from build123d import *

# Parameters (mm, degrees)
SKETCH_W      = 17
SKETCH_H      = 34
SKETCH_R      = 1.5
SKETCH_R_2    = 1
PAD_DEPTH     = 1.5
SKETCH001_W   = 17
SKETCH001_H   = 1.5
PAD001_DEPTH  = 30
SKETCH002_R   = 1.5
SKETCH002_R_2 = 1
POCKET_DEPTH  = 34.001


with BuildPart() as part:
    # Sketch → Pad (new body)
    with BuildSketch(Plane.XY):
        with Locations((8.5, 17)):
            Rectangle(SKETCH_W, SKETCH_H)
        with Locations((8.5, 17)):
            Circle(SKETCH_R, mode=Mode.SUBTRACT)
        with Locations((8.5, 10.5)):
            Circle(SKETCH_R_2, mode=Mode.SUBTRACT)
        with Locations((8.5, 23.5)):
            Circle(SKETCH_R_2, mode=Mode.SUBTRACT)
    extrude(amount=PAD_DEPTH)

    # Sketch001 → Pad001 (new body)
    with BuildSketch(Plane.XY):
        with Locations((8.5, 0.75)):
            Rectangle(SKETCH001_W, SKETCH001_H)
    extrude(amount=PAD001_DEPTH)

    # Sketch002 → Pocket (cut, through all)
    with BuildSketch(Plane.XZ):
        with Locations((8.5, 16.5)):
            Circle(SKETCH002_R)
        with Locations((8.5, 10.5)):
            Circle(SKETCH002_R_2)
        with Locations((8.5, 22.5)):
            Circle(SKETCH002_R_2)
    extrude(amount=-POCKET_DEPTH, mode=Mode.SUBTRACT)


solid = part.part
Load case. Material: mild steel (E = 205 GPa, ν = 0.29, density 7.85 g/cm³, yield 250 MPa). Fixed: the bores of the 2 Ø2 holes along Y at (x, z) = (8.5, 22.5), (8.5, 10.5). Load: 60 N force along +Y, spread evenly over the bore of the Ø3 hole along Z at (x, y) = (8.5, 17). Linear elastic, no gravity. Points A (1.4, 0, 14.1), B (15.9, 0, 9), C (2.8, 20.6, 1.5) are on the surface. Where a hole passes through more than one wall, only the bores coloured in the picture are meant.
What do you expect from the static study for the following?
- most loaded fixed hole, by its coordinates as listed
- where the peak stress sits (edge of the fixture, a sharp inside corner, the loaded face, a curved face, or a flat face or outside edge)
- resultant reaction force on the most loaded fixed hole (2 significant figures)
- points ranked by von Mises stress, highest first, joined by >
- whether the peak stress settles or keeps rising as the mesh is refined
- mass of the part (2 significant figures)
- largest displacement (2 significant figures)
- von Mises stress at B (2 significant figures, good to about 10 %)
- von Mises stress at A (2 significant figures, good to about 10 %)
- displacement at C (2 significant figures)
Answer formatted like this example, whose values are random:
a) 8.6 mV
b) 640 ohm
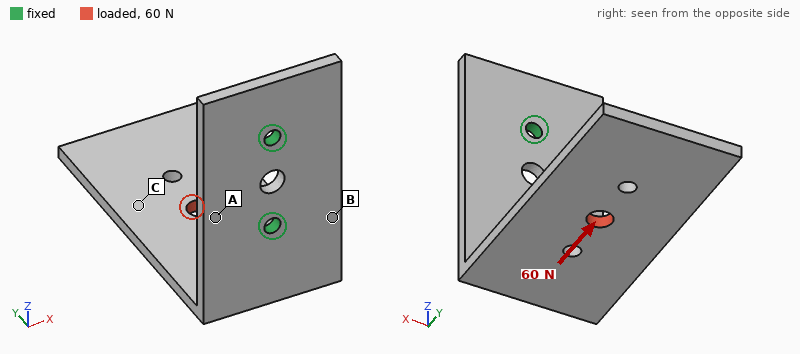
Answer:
a) (8.5, 10.5)
b) edge of the fixture
c) 76 N
d) B > A > C
e) keeps rising
f) 12 g
g) 0.11 mm
h) 46 MPa
i) 20 MPa
j) 0.065 mm
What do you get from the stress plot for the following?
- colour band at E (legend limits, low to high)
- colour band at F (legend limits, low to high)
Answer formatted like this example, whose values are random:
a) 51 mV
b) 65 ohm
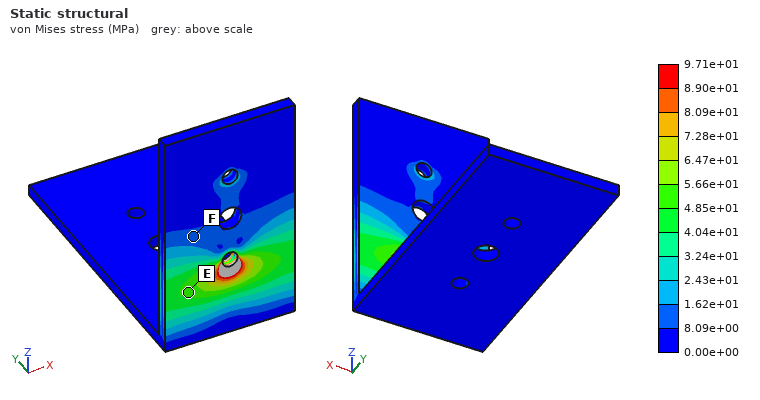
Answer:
a) 4.85e+01 to 5.66e+01 MPa
b) 8.09e+00 to 1.62e+01 MPa
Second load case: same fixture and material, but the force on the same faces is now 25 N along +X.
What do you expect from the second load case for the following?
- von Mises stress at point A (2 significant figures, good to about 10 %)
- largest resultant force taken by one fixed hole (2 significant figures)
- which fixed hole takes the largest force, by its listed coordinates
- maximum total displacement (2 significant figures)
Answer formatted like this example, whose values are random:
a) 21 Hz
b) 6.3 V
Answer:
a) 26 MPa
b) 41 N
c) (8.5, 10.5)
d) 83 µm
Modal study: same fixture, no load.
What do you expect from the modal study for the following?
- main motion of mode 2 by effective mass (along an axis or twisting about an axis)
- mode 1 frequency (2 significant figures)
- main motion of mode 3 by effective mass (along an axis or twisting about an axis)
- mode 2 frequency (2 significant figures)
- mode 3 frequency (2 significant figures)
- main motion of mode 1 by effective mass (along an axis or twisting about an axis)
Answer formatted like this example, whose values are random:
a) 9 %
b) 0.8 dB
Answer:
a) along X
b) 760 Hz
c) along Y
d) 1300 Hz
e) 3700 Hz
f) along Z
